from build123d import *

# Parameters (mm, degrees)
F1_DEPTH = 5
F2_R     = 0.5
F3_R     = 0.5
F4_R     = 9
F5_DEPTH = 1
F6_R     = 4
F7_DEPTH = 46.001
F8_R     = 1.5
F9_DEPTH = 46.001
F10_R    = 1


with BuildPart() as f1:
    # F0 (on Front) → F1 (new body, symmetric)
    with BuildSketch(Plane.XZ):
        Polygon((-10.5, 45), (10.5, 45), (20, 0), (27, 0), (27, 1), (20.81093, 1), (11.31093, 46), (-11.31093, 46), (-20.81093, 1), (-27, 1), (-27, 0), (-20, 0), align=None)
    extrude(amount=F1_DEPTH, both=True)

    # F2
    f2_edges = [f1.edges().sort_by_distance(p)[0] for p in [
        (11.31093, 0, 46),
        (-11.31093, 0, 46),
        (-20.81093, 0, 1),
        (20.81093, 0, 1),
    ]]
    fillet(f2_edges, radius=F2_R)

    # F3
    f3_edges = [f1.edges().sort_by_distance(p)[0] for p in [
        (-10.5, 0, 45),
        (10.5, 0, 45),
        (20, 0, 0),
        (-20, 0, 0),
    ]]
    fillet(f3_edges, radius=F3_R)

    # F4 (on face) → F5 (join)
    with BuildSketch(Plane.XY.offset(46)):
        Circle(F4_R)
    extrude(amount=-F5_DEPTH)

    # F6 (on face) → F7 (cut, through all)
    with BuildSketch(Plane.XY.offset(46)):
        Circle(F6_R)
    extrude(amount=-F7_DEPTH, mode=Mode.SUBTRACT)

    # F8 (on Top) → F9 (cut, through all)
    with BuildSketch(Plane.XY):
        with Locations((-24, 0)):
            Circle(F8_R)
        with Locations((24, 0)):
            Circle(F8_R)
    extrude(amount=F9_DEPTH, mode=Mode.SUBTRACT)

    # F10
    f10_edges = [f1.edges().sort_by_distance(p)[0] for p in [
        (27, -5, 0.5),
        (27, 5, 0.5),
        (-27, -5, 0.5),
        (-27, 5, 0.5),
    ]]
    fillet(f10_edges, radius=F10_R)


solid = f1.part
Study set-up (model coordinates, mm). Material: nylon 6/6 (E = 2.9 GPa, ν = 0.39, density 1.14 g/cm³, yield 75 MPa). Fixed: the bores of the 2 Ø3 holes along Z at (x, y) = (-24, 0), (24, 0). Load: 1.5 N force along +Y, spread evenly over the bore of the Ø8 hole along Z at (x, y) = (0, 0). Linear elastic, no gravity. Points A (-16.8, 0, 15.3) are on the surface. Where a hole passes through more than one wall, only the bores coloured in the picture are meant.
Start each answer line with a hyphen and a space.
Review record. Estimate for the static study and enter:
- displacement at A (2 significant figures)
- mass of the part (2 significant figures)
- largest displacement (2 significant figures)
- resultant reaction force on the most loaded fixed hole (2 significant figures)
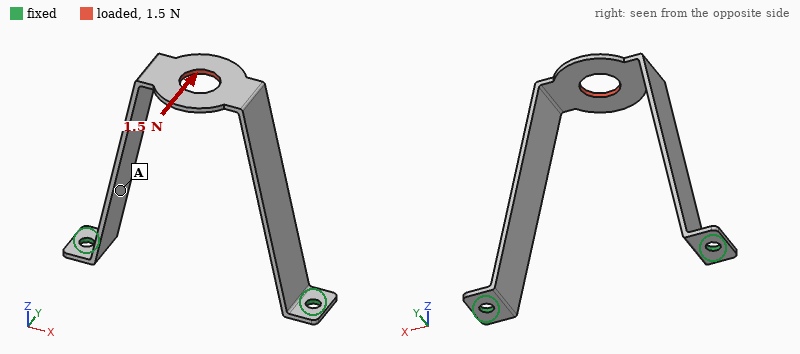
- 0.23 mm
- 1.5 g
- 0.78 mm
- 0.75 N
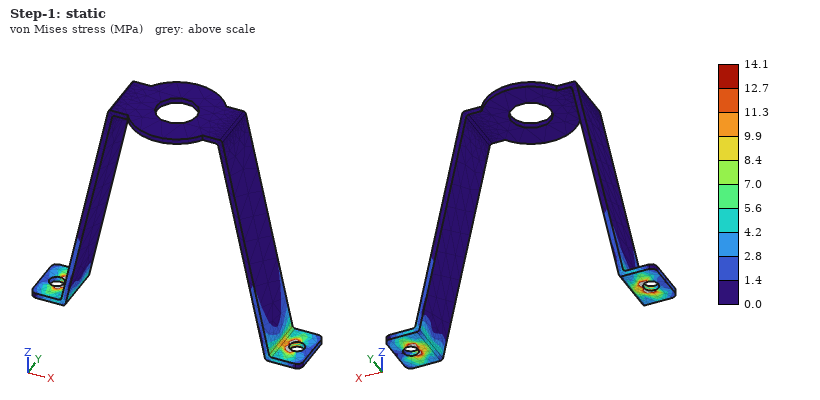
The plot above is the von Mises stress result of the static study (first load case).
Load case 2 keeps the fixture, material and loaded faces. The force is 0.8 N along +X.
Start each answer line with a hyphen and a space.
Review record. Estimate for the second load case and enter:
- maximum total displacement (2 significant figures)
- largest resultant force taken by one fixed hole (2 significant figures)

- 0.78 mm
- 0.73 N
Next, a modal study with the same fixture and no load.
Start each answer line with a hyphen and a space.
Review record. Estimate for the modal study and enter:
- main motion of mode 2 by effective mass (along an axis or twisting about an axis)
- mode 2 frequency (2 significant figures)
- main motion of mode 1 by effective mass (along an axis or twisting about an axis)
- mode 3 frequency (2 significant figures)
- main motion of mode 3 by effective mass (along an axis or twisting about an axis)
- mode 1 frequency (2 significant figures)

- along Y
- 280 Hz
- along X
- 460 Hz
- twisting about Z
- 180 Hz
